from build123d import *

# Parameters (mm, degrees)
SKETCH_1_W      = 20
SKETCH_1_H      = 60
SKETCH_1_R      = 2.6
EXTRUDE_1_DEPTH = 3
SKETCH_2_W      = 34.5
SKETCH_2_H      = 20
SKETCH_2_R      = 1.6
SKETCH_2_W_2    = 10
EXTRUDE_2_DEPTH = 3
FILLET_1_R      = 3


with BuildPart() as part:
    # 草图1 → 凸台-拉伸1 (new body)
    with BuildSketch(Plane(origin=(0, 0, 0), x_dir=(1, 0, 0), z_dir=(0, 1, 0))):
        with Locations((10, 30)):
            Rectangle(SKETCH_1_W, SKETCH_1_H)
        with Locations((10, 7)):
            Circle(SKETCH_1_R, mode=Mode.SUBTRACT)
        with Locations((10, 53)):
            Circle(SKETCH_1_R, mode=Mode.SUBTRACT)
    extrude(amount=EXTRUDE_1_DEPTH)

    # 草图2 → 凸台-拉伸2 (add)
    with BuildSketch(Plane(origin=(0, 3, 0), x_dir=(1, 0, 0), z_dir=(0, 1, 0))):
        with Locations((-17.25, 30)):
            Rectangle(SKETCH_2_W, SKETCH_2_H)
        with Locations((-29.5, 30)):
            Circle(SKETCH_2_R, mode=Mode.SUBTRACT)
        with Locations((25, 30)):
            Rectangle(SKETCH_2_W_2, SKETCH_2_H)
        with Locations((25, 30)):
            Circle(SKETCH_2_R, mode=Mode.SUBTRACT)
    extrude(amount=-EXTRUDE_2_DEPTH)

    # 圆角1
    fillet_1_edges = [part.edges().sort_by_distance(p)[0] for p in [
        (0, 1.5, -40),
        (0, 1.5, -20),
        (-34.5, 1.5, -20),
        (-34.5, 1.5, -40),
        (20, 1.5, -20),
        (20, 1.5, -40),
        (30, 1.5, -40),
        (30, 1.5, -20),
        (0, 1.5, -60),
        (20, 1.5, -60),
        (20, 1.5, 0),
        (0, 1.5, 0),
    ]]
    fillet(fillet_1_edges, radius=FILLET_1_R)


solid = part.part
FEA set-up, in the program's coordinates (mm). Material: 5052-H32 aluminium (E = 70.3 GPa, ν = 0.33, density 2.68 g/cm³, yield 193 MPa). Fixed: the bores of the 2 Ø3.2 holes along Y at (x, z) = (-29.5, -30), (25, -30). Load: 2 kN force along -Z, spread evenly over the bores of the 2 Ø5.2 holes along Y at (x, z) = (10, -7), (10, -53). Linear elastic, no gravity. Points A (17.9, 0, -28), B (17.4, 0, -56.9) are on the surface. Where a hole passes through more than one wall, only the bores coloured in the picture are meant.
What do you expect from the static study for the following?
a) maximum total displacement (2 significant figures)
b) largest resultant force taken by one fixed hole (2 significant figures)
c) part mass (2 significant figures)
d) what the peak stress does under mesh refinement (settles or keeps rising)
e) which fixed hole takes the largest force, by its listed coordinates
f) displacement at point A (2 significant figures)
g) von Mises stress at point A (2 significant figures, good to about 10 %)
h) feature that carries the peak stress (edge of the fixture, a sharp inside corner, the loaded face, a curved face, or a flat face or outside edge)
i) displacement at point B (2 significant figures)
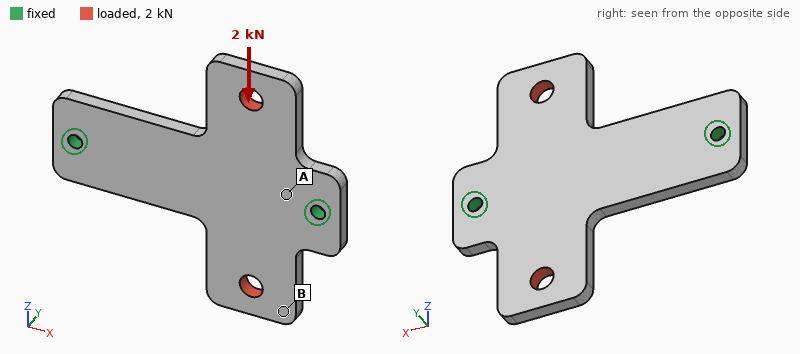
37 µm
1.5 kN
16 g
keeps rising
(25, -30)
12 µm
30 MPa
edge of the fixture
27 µm
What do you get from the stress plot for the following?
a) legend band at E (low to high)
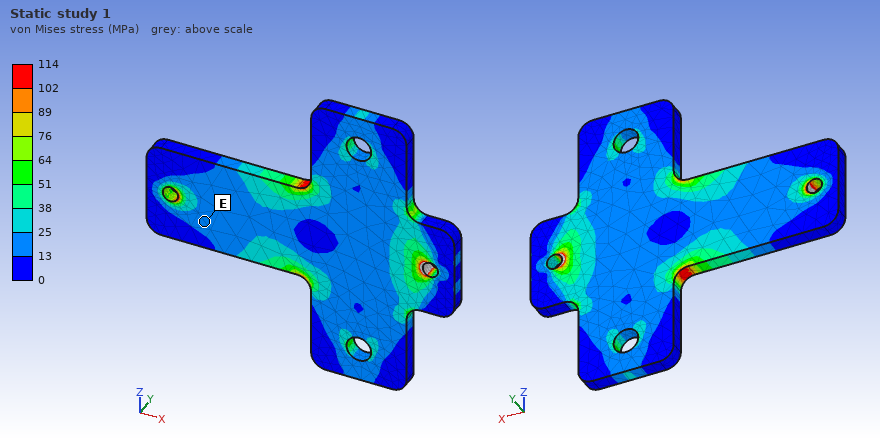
13 to 25 MPa
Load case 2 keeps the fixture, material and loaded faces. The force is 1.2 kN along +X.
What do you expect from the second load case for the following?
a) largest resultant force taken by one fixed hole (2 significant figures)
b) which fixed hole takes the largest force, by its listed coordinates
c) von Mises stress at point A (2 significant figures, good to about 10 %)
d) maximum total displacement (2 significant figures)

800 N
(25, -30)
12 MPa
21 µm
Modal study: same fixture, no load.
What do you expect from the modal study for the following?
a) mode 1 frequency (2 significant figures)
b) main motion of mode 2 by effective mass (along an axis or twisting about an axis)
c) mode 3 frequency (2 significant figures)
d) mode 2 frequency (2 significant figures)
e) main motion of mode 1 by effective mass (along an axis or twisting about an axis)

2200 Hz
along Y
5500 Hz
2900 Hz
twisting about X
